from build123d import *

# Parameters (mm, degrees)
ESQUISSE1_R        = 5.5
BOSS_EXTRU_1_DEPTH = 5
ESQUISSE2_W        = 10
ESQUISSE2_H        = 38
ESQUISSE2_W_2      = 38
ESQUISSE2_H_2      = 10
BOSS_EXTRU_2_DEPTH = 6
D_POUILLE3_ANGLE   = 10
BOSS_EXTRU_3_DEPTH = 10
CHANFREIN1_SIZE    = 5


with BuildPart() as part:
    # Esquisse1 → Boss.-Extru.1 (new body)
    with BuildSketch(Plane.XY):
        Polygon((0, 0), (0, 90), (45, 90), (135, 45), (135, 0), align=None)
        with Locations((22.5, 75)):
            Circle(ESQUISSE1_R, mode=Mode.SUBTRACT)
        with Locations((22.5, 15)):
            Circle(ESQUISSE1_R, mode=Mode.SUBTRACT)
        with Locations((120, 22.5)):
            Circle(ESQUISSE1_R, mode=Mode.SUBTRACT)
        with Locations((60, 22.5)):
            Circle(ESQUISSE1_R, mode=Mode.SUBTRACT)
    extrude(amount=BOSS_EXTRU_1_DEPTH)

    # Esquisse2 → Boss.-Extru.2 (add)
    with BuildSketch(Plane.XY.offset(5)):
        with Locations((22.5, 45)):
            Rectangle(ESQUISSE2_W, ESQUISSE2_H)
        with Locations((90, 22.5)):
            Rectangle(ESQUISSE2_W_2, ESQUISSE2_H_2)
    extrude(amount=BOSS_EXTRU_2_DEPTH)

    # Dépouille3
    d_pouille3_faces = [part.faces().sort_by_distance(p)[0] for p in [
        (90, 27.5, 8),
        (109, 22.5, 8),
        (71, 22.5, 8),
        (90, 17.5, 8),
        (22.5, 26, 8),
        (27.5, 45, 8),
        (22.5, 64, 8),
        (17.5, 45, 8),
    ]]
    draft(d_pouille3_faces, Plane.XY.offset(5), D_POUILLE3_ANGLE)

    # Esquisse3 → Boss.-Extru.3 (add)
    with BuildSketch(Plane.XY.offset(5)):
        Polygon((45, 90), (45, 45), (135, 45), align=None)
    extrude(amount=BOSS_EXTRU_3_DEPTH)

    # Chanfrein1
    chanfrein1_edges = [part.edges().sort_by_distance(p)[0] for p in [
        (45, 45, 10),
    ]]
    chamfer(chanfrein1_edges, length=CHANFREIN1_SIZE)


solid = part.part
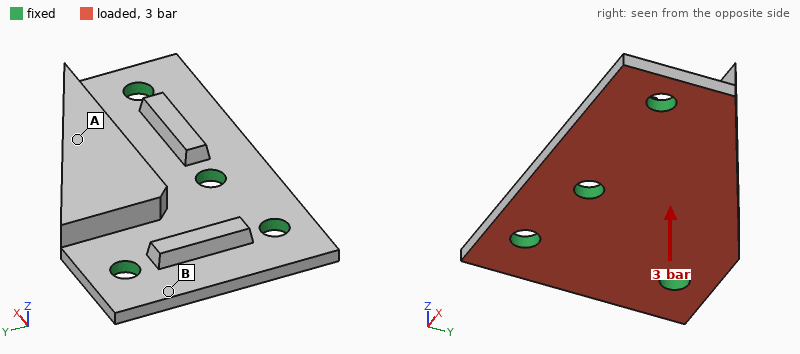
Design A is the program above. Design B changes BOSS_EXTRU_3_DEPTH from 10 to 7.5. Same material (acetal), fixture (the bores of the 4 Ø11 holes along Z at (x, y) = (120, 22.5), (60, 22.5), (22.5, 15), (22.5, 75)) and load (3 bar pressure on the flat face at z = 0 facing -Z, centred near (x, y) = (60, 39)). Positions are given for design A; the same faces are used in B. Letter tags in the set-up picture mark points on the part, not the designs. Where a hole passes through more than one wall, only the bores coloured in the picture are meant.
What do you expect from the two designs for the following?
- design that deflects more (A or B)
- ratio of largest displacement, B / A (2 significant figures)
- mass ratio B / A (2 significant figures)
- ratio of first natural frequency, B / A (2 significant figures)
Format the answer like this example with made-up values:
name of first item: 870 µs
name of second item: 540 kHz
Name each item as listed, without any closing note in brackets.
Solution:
design that deflects more: B
ratio of largest displacement, B / A: 1.2
mass ratio B / A: 0.93
ratio of first natural frequency, B / A: 1.0
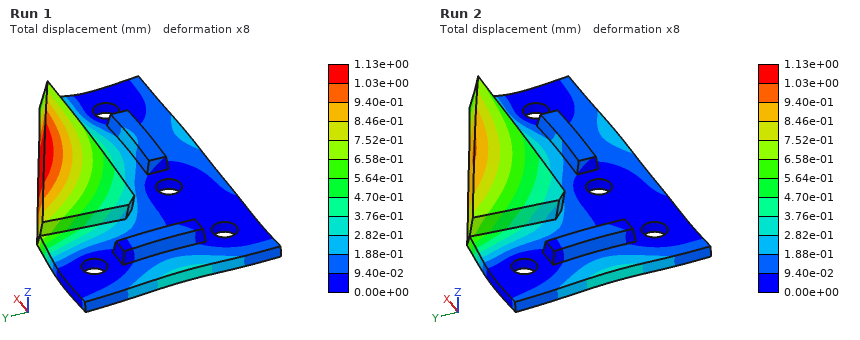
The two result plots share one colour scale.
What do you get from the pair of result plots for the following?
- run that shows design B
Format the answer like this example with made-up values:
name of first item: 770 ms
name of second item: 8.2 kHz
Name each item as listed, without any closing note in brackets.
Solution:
run that shows design B: Run 1
